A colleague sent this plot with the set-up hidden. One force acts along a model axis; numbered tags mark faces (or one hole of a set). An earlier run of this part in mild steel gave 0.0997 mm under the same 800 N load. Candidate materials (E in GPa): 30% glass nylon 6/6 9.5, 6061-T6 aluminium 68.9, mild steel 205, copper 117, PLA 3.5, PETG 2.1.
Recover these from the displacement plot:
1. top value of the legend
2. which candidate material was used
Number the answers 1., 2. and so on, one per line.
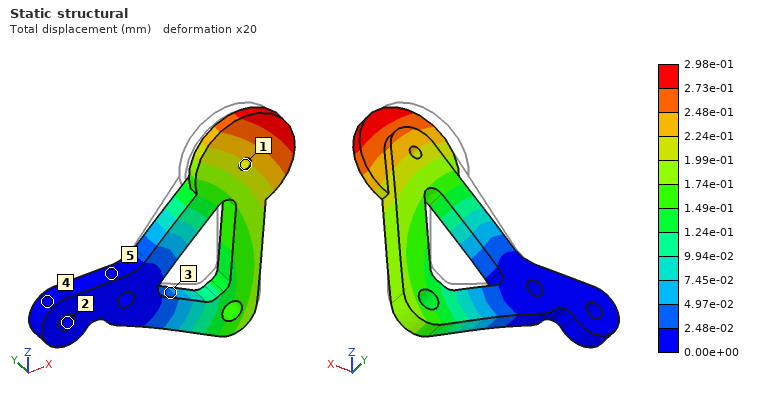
1. 2.98e-01 mm
2. 6061-T6 aluminium
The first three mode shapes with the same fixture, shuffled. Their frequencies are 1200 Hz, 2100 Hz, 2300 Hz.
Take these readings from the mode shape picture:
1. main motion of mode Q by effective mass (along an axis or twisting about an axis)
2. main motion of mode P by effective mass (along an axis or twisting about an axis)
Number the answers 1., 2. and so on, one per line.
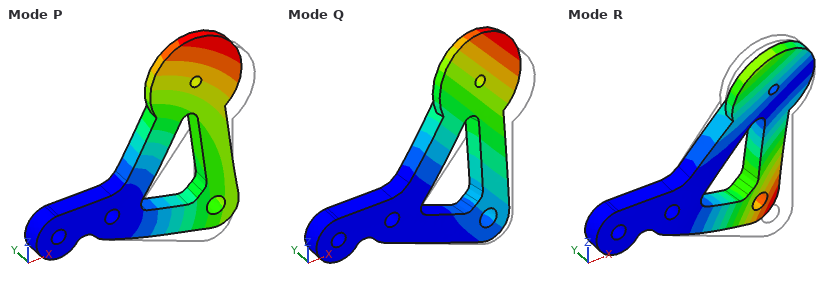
1. along Y
2. along Z
